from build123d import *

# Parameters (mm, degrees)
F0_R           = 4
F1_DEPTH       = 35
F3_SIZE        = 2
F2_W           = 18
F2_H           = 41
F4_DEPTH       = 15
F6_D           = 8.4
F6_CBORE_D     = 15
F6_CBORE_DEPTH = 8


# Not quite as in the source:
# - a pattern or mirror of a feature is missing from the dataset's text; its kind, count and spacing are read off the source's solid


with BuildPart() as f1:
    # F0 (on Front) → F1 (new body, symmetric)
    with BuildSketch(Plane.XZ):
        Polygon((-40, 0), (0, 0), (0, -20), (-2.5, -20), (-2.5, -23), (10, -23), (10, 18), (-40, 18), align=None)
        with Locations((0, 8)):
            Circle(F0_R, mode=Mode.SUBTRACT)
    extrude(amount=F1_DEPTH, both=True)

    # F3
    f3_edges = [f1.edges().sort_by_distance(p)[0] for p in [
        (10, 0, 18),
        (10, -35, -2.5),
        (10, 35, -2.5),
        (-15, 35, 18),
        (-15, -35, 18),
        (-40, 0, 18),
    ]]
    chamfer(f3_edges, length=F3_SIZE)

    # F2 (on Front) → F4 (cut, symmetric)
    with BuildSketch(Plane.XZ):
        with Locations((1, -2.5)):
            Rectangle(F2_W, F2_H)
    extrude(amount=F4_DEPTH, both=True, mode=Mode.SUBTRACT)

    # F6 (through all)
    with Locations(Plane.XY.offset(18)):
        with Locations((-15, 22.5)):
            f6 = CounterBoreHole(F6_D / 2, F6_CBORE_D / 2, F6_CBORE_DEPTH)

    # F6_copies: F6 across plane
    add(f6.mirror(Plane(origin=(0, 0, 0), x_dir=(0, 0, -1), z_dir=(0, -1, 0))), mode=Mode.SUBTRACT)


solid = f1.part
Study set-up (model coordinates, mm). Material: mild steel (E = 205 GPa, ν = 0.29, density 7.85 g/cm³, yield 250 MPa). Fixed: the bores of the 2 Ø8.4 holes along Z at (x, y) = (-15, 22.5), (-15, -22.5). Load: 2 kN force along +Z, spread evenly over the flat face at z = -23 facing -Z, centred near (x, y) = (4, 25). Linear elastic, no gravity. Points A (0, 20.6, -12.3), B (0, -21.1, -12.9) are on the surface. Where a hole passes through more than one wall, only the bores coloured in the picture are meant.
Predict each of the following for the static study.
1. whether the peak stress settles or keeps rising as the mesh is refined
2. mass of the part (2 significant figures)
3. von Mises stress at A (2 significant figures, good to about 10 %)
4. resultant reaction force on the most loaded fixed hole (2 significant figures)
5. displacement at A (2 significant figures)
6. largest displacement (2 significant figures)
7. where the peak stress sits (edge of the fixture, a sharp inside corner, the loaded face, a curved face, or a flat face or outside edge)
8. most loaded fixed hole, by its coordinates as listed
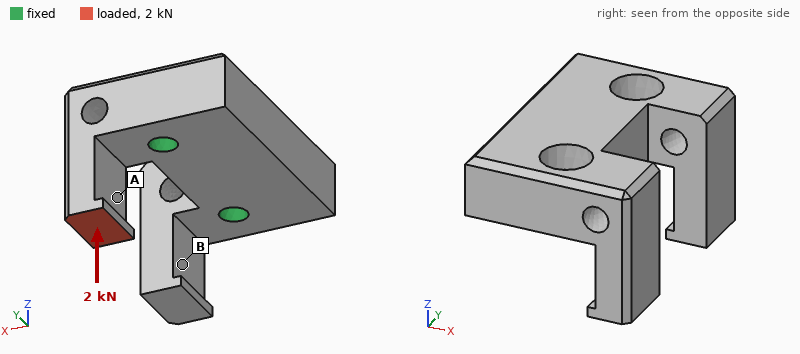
keeps rising
440 g
18 MPa
2.1 kN
11 µm
16 µm
edge of the fixture
(-15, 22.5)
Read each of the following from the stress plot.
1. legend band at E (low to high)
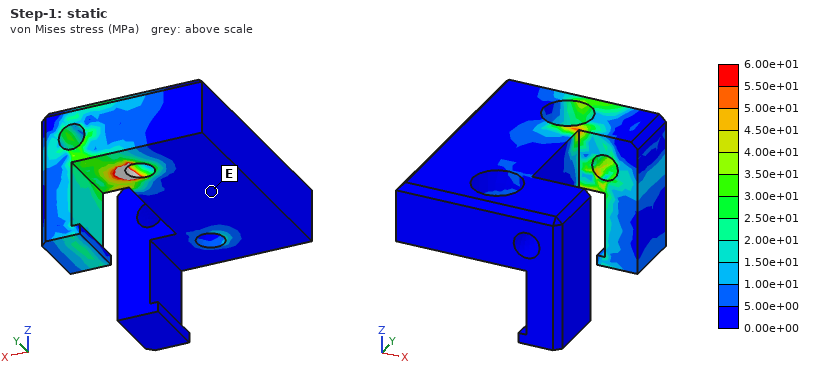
0.00e+00 to 5.00e+00 MPa
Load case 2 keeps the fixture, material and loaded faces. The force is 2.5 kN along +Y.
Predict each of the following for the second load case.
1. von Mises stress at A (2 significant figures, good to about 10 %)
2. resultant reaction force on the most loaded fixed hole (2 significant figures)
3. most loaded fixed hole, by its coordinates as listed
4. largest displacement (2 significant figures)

42 MPa
3.4 kN
(-15, 22.5)
75 µm
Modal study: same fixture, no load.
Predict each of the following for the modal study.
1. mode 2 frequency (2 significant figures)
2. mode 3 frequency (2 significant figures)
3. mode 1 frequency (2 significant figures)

6000 Hz
6900 Hz
5600 Hz
